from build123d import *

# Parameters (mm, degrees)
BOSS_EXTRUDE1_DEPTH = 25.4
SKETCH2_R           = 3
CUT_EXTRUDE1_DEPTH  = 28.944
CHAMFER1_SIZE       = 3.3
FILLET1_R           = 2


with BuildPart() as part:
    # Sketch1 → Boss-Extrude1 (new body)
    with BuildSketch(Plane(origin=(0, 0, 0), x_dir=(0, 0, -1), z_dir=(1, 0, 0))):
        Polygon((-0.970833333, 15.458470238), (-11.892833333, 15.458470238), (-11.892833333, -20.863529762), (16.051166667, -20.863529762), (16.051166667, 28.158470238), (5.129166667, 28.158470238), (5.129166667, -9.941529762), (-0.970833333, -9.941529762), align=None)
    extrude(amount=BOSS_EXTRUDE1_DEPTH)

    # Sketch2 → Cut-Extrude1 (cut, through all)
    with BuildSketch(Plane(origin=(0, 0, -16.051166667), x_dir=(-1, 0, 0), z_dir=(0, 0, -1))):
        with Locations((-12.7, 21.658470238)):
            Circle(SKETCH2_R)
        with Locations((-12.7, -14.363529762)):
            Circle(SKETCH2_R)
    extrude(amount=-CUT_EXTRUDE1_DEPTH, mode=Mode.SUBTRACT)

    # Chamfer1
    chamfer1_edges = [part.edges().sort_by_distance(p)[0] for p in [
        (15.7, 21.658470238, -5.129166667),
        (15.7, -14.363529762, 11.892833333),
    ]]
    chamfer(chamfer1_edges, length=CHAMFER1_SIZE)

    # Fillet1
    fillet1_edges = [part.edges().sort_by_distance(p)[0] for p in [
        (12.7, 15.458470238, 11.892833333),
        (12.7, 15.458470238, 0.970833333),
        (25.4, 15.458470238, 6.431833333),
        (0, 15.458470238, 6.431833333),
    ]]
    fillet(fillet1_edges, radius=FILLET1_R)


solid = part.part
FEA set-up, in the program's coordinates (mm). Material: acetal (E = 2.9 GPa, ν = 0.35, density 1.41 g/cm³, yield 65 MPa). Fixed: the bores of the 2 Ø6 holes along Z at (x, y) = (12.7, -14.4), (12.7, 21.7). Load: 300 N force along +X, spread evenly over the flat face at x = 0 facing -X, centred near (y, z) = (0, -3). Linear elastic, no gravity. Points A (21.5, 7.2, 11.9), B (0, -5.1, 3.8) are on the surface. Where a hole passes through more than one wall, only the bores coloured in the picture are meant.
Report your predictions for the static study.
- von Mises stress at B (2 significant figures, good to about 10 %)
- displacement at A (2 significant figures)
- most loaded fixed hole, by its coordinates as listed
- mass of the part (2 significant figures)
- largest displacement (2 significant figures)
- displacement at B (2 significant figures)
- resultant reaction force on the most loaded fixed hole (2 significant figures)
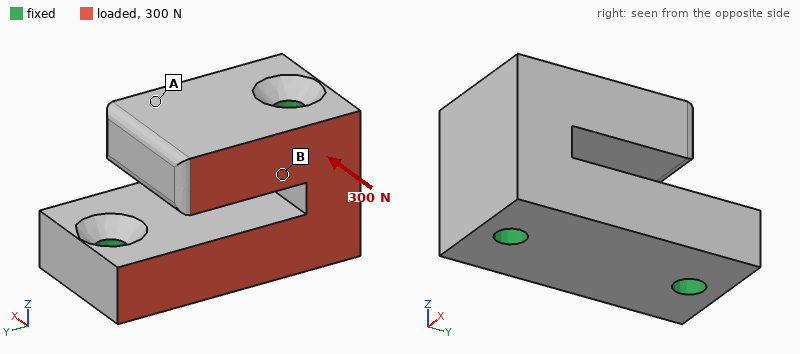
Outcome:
0.78 MPa
21 µm
(12.7, -14.4)
34 g
30 µm
14 µm
210 N
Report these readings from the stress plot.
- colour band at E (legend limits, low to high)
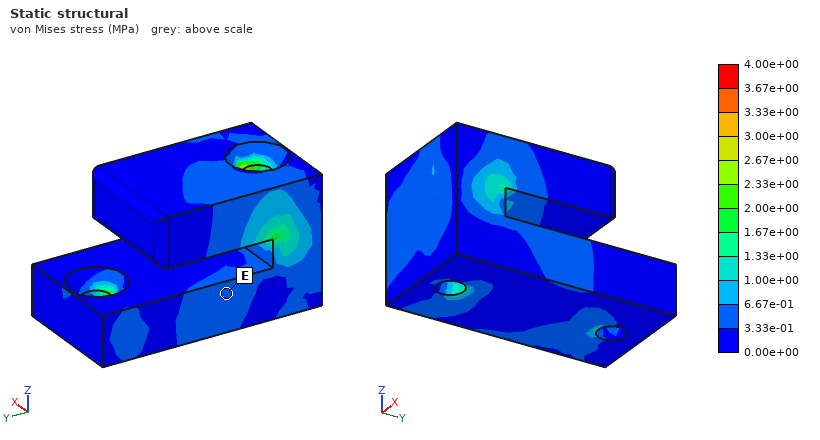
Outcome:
3.33e-01 to 6.67e-01 MPa
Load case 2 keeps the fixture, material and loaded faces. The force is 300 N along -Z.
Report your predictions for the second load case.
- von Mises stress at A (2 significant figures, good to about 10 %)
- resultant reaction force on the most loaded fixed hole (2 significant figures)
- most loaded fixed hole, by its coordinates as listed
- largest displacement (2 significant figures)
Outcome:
0.53 MPa
220 N
(12.7, -14.4)
69 µm
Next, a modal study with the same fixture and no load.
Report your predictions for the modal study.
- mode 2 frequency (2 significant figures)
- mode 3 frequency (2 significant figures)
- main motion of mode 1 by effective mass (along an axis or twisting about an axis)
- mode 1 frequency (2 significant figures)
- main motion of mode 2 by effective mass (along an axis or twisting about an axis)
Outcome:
2900 Hz
5200 Hz
along Z
2400 Hz
along X
